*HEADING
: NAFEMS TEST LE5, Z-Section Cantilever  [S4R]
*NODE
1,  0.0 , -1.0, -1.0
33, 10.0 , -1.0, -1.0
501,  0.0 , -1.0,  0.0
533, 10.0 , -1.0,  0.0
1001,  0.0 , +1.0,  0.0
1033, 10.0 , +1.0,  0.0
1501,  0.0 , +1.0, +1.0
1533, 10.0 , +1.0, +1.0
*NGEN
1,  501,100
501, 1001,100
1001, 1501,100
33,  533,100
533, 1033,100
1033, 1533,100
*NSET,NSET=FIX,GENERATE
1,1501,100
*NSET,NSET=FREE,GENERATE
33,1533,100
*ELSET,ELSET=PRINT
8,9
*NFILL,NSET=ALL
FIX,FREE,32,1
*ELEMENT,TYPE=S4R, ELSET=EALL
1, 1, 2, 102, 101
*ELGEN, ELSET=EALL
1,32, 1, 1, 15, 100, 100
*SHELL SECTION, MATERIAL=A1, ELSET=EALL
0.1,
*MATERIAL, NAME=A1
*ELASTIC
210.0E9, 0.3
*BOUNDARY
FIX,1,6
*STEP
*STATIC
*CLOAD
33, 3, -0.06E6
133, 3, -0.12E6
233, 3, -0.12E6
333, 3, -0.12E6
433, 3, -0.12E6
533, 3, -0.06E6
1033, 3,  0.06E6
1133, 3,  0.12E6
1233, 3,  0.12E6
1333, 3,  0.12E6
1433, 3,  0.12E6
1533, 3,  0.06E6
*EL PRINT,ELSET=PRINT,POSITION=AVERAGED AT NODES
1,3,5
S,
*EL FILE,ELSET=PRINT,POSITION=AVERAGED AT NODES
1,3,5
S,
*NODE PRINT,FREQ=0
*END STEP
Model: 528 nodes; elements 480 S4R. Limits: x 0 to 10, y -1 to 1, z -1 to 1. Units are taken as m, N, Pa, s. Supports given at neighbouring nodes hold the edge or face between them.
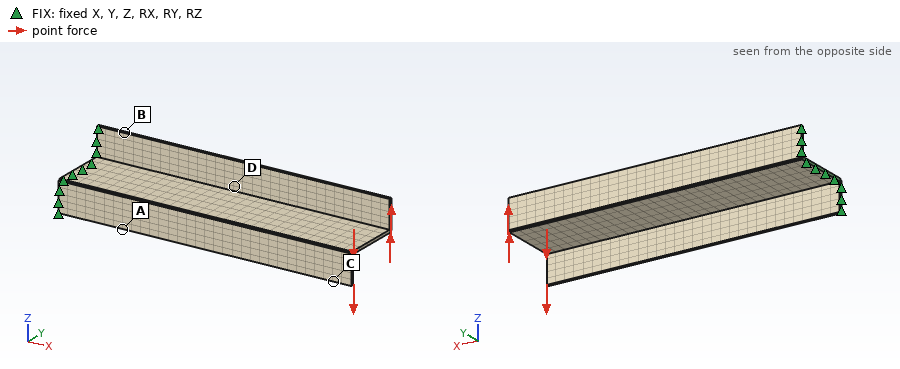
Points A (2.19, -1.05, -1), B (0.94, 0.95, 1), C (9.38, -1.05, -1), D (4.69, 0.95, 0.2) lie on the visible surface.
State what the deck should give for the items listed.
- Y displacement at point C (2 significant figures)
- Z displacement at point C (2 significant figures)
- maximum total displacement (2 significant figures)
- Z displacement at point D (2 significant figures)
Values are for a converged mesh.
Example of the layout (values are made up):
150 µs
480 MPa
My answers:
0.027 m
-0.031 m
0.044 m
0.0089 m
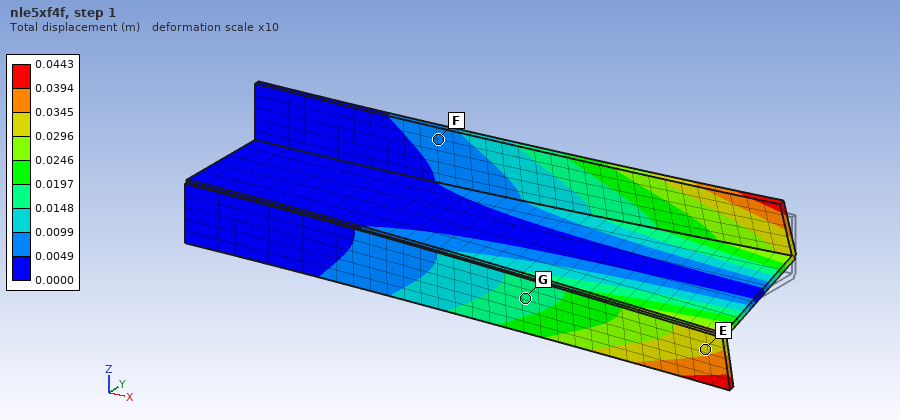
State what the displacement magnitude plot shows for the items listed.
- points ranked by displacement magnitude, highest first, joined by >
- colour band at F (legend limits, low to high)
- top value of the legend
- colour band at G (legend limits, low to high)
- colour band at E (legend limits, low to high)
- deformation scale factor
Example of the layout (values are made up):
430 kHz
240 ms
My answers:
E > G > F
0.0049 to 0.0099 m
0.0443 m
0.0148 to 0.0197 m
0.0296 to 0.0345 m
10
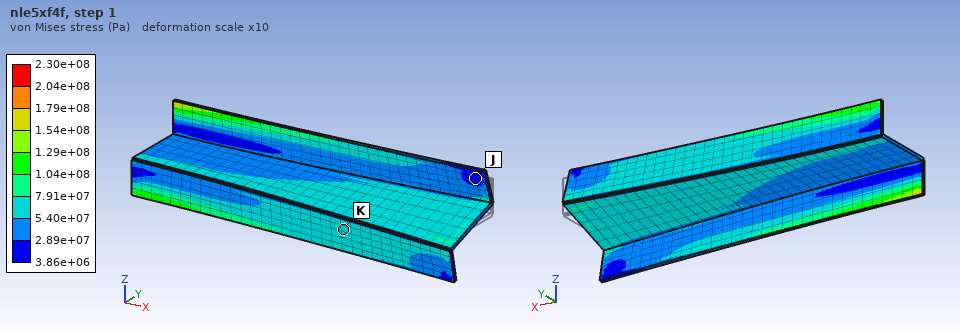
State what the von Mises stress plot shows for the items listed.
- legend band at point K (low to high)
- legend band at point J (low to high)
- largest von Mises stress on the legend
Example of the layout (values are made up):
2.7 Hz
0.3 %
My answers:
5.40e+07 to 7.91e+07 Pa
3.86e+06 to 2.89e+07 Pa
2.30e+08 Pa
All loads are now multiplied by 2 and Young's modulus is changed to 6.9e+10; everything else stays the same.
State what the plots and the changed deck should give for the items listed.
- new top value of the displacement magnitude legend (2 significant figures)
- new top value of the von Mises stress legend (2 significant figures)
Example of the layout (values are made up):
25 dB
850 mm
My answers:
0.27 m
4.6e+08 Pa
